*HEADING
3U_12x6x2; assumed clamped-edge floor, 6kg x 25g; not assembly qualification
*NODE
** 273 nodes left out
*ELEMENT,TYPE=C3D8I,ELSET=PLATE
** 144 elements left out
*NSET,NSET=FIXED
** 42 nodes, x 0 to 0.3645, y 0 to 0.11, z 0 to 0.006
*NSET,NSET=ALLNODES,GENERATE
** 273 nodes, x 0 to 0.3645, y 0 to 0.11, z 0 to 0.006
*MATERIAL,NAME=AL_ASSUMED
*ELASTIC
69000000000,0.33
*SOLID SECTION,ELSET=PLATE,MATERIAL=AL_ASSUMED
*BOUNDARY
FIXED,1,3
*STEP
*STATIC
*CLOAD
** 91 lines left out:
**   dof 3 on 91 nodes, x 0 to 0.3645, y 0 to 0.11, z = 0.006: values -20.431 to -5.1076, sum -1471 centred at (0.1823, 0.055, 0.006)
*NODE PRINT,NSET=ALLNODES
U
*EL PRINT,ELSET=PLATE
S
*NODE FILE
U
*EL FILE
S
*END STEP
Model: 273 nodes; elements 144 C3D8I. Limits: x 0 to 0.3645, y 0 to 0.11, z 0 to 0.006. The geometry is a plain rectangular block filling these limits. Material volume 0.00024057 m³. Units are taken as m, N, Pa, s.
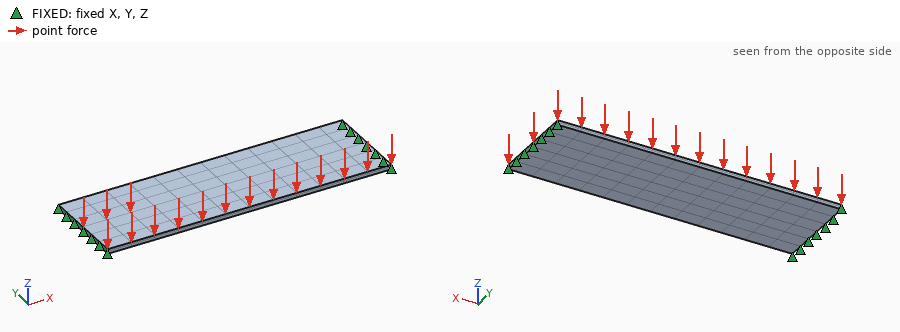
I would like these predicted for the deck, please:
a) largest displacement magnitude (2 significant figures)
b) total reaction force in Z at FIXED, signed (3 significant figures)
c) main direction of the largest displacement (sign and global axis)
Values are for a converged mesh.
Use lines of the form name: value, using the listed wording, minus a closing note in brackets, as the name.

largest displacement magnitude: 0.0013 m
total reaction force in Z at FIXED, signed: 1470 N
main direction of the largest displacement: -Z
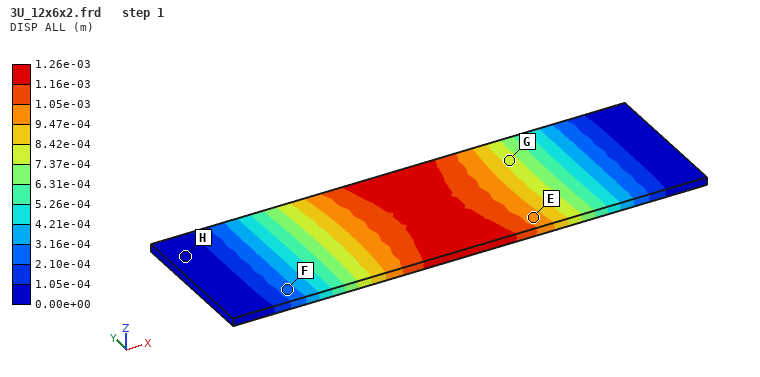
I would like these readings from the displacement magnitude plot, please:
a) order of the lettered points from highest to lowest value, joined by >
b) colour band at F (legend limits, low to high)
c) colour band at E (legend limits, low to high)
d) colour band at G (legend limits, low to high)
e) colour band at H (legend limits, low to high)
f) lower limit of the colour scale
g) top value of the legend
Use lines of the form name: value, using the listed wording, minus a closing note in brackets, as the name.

order of the lettered points from highest to lowest value, joined by >: E > G > F > H
colour band at F: 2.10e-04 to 3.16e-04 m
colour band at E: 9.47e-04 to 1.05e-03 m
colour band at G: 7.37e-04 to 8.42e-04 m
colour band at H: 0.00e+00 to 1.05e-04 m
lower limit of the colour scale: 0.00e+00 m
top value of the legend: 1.26e-03 m
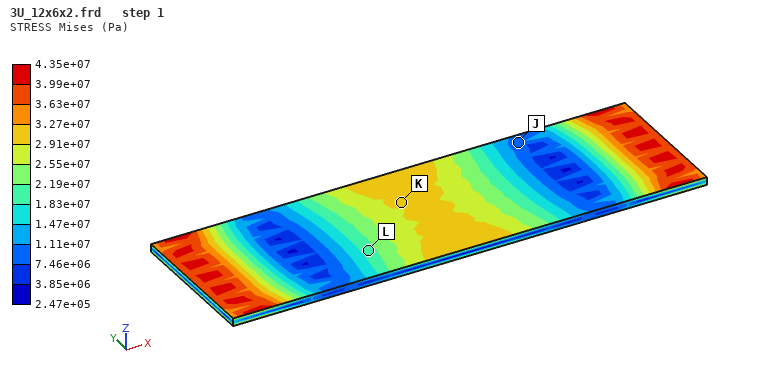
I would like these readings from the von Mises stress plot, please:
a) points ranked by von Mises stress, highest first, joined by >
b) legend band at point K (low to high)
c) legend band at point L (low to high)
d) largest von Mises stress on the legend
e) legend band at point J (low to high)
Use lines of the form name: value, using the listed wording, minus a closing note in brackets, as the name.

points ranked by von Mises stress, highest first, joined by >: K > L > J
legend band at point K: 2.91e+07 to 3.27e+07 Pa
legend band at point L: 1.83e+07 to 2.19e+07 Pa
largest von Mises stress on the legend: 4.35e+07 Pa
legend band at point J: 7.46e+06 to 1.11e+07 Pa
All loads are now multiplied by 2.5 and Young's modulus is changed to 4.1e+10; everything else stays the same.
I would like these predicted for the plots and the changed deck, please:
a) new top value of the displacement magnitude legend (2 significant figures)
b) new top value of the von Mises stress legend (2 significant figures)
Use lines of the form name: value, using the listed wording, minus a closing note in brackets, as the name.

new top value of the displacement magnitude legend: 0.0053 m
new top value of the von Mises stress legend: 1.1e+08 Pa
